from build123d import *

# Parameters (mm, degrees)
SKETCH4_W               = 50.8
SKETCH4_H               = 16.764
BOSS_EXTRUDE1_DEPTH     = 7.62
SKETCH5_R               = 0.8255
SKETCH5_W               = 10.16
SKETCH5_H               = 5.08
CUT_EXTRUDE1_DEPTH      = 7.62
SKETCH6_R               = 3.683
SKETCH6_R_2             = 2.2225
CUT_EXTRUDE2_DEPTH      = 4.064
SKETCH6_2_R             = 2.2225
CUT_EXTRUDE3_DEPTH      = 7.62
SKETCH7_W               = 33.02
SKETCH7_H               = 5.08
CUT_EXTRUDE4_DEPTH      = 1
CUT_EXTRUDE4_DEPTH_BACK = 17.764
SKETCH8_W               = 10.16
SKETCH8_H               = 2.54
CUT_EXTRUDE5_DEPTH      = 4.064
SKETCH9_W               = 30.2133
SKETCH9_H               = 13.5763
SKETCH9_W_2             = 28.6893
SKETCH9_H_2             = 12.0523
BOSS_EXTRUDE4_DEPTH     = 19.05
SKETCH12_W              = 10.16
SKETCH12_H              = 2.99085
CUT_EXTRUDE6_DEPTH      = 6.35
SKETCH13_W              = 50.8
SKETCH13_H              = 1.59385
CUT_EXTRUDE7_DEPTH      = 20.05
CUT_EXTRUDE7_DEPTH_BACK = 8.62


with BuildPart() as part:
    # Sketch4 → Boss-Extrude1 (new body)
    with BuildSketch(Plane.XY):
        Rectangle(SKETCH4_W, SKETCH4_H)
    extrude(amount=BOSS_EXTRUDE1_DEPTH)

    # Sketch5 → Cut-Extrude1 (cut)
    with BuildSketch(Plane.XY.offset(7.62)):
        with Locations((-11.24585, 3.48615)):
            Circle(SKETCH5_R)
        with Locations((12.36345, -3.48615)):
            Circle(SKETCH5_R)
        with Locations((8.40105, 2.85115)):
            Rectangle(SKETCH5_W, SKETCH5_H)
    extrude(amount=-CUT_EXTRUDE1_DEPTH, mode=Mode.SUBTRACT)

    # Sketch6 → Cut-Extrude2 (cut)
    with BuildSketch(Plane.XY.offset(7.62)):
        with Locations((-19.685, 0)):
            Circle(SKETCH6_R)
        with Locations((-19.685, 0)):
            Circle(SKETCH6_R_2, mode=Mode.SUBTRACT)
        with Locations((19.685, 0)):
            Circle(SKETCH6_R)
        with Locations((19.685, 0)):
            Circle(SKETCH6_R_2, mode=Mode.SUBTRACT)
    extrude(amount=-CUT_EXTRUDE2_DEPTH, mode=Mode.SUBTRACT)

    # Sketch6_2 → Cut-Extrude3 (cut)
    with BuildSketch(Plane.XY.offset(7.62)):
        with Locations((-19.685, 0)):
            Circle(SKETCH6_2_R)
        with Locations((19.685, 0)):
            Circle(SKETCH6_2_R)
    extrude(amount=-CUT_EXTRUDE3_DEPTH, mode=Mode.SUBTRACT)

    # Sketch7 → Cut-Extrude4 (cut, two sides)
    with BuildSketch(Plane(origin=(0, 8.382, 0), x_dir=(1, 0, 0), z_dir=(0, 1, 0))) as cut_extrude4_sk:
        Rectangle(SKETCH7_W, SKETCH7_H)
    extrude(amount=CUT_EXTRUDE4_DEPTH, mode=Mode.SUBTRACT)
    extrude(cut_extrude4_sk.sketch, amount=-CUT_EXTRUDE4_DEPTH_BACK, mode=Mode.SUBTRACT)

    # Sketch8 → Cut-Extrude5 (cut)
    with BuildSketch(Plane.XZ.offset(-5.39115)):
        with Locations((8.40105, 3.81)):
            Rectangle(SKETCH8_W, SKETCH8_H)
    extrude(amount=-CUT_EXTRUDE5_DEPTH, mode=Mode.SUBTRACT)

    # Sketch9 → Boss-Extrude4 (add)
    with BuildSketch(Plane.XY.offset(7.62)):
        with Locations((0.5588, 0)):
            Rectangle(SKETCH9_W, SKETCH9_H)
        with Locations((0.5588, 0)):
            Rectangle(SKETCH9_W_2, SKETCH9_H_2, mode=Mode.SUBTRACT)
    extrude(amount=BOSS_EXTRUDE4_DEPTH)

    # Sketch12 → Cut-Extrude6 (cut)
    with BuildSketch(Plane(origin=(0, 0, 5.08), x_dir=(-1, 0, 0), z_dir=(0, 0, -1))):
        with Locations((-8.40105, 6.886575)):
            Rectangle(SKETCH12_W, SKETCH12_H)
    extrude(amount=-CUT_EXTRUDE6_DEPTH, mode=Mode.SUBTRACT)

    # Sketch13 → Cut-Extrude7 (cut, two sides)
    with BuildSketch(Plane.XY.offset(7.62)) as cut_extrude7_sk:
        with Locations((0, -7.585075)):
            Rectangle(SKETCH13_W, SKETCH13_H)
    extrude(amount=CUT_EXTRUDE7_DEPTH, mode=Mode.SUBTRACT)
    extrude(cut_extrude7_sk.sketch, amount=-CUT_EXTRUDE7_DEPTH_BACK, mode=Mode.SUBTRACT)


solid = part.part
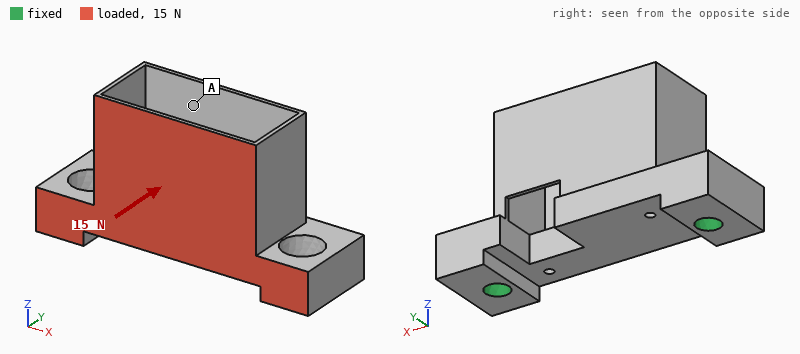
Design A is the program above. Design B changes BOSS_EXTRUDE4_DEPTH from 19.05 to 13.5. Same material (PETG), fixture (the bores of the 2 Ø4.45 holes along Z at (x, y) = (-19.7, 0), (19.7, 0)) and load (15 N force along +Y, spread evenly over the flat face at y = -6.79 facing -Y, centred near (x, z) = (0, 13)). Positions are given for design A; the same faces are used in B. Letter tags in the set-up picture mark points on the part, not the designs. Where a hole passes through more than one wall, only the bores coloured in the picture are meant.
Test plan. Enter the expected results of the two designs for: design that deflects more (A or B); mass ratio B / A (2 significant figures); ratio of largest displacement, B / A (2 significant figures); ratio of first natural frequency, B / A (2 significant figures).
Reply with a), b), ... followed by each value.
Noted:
a) A
b) 0.93
c) 0.75
d) 1.3
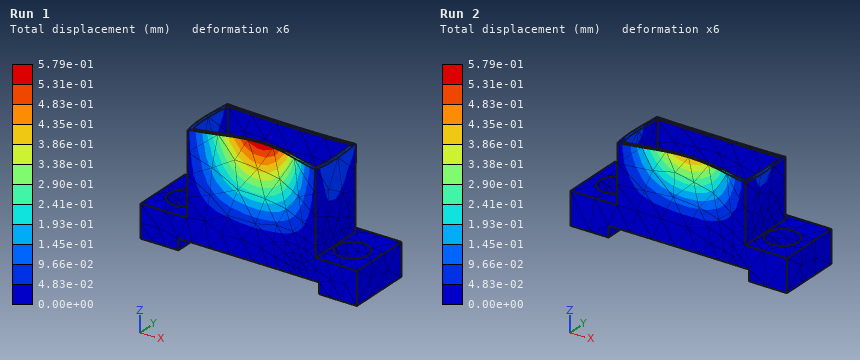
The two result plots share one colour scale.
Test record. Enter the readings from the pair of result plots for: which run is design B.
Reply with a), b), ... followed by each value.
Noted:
a) Run 2
